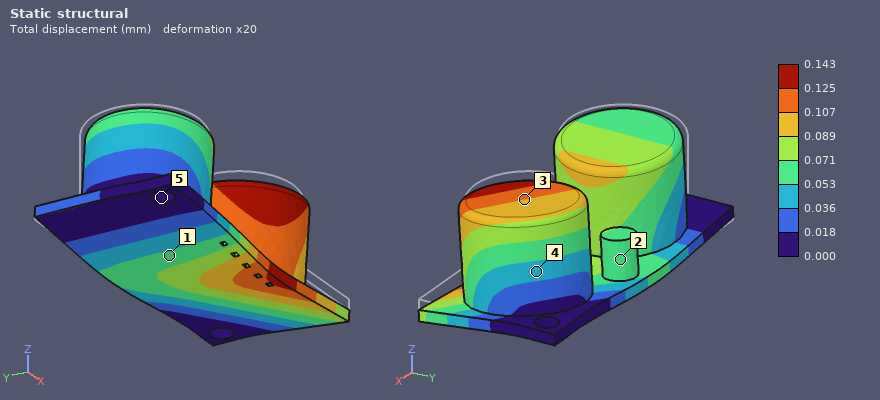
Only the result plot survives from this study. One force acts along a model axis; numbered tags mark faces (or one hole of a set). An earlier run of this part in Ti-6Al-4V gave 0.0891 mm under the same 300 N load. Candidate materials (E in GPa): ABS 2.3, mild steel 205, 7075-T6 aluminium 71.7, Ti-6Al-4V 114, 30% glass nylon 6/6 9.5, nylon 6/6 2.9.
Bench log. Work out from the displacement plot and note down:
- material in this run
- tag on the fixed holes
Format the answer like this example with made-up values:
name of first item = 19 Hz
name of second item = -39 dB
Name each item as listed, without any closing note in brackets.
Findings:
material in this run = 7075-T6 aluminium
tag on the fixed holes = 5
